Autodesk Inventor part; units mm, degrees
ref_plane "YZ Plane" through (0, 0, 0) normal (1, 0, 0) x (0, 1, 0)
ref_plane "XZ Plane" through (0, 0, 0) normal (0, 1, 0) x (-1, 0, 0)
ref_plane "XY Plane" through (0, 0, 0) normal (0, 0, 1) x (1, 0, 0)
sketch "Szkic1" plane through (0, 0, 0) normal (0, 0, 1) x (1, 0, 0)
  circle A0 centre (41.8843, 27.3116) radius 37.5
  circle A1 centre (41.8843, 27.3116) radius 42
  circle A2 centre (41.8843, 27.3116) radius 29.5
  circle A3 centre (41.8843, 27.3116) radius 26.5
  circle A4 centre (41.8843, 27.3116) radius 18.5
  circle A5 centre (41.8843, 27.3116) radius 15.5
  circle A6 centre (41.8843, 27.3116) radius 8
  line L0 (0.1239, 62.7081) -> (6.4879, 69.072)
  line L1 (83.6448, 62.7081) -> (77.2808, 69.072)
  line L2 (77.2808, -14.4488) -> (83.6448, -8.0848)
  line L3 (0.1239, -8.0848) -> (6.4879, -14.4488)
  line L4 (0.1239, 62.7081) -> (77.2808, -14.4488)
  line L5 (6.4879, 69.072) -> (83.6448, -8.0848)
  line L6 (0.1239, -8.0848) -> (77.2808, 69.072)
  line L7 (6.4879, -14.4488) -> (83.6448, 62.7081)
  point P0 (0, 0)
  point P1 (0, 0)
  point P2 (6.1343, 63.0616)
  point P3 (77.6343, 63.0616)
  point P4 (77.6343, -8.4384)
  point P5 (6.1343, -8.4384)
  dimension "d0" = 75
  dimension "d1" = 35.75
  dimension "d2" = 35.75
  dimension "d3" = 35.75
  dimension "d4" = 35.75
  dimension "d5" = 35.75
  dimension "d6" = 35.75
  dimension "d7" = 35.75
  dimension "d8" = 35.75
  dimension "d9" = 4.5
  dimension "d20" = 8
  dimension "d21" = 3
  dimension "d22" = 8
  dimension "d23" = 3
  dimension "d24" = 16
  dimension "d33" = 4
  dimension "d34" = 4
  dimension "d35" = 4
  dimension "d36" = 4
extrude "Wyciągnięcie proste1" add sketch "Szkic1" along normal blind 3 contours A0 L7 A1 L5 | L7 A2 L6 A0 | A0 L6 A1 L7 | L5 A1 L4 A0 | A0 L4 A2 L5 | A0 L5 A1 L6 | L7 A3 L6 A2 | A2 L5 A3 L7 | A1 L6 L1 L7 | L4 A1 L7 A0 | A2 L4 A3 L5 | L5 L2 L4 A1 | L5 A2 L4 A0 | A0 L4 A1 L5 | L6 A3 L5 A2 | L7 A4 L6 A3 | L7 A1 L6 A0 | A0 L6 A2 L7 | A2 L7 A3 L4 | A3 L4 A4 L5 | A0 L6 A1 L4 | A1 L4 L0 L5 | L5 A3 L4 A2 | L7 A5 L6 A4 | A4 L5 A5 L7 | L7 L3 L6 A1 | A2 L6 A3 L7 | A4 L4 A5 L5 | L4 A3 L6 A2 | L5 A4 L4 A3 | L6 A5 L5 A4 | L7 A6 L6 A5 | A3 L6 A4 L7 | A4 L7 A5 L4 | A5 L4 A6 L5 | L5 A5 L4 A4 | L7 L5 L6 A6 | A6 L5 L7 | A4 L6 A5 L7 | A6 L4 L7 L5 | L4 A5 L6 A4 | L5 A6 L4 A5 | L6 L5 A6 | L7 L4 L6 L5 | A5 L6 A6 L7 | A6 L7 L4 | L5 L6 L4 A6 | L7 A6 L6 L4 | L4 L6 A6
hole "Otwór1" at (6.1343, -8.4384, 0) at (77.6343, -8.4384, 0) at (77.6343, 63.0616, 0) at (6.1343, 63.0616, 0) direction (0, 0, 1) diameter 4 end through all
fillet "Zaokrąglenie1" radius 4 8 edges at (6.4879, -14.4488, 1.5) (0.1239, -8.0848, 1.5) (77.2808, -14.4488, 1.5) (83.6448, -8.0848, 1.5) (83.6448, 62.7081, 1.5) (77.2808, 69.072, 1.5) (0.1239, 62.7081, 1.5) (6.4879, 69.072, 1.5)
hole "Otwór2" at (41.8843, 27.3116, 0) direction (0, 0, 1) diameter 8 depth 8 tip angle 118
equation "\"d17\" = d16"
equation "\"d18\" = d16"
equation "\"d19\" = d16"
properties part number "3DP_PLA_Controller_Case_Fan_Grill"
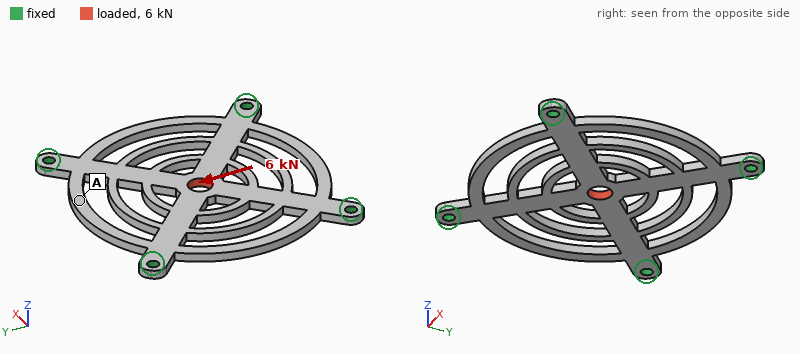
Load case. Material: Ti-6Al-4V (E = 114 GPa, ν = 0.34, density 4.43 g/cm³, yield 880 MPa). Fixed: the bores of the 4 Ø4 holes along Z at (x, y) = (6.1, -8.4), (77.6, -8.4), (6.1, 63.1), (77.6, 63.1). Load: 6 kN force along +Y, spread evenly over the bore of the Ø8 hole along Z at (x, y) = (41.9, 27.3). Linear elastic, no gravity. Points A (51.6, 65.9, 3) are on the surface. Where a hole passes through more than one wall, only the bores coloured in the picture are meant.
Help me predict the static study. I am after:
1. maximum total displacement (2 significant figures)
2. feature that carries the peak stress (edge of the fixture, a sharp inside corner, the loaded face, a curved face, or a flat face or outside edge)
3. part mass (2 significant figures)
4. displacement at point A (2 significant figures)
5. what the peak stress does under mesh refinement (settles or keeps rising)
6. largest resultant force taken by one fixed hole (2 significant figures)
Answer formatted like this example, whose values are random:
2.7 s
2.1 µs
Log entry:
47 µm
edge of the fixture
45 g
8.9 µm
keeps rising
2.0 kN
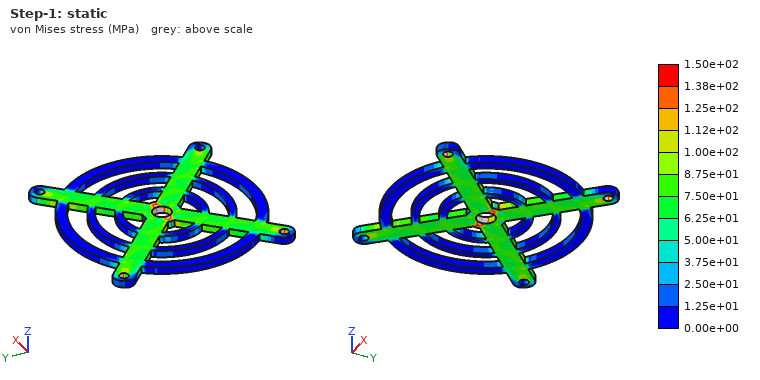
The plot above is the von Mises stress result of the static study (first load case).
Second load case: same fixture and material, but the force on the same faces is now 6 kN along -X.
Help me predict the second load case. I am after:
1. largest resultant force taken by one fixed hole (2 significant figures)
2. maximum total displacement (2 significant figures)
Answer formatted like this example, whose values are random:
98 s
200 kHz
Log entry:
2.0 kN
47 µm
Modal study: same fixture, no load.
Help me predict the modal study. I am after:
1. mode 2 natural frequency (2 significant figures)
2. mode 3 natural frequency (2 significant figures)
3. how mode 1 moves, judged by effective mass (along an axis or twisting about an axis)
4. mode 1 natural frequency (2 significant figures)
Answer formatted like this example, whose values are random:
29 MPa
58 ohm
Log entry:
3100 Hz
3100 Hz
along Z
1800 Hz
